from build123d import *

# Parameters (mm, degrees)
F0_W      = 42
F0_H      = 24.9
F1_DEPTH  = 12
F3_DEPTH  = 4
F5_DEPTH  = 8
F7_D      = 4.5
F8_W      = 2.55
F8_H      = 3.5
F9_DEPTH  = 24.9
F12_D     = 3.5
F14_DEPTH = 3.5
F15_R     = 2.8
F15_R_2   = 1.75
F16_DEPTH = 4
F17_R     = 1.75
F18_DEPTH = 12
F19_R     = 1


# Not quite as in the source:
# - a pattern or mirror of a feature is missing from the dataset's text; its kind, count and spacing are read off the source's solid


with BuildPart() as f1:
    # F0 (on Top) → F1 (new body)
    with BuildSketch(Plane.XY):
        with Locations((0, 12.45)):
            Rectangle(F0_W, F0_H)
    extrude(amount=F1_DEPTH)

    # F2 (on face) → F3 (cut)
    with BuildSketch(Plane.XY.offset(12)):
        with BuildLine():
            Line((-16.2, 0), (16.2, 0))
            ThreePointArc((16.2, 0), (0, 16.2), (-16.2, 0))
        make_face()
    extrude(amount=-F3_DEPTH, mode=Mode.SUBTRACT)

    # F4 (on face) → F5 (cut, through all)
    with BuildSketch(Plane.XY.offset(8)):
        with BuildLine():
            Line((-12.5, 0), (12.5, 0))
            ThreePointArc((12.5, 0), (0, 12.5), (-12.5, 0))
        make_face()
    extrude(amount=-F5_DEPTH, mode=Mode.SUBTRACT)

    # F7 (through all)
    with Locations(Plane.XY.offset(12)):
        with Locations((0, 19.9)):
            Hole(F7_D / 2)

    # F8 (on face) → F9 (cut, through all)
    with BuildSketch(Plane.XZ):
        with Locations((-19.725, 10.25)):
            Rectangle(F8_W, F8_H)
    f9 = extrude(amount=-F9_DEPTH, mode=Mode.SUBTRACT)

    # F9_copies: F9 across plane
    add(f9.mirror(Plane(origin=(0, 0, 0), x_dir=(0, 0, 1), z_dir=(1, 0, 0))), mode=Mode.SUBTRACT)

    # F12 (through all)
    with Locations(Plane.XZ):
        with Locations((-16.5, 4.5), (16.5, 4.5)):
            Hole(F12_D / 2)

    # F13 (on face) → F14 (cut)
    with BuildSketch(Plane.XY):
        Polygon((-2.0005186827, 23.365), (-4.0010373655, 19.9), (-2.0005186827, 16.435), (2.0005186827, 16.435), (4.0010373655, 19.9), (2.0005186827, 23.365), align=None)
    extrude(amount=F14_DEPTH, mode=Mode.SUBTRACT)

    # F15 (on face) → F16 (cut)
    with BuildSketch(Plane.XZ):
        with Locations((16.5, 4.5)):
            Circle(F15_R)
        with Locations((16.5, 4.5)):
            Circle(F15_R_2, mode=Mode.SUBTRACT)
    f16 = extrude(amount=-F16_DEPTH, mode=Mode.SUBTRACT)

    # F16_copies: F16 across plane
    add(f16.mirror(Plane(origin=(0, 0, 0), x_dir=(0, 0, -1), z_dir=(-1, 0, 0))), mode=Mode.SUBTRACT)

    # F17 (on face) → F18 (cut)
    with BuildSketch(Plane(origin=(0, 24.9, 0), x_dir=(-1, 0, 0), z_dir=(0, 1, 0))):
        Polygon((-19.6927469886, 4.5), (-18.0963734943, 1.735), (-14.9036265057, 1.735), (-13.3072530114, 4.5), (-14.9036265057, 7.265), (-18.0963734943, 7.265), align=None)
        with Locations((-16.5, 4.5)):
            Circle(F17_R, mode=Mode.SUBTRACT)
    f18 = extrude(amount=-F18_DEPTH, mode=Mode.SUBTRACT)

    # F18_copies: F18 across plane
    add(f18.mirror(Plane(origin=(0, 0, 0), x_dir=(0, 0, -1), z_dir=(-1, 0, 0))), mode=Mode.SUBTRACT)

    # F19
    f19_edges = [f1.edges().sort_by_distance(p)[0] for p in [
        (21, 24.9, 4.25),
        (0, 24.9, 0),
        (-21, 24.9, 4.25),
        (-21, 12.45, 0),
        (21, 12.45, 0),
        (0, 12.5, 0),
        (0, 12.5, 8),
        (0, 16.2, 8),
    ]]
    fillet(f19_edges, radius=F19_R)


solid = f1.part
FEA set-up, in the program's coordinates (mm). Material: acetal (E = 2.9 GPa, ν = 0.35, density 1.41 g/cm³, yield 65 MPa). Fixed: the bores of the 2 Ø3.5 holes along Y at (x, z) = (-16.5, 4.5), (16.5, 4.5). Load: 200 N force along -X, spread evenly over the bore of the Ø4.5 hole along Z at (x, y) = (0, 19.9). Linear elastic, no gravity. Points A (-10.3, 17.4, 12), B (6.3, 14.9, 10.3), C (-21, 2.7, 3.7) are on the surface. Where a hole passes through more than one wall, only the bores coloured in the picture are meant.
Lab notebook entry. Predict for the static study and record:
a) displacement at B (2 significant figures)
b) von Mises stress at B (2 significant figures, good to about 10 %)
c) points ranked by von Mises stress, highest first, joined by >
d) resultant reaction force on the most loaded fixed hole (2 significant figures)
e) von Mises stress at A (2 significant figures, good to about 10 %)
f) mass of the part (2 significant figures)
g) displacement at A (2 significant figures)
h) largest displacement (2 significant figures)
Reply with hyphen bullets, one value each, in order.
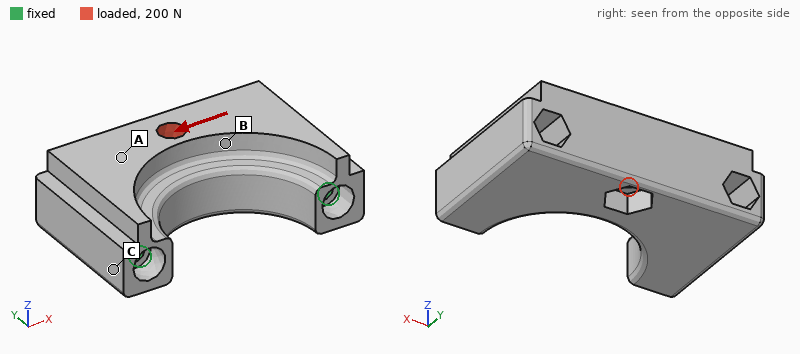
- 9.7 µm
- 2.0 MPa
- B > A > C
- 110 N
- 0.96 MPa
- 10 g
- 10 µm
- 16 µm
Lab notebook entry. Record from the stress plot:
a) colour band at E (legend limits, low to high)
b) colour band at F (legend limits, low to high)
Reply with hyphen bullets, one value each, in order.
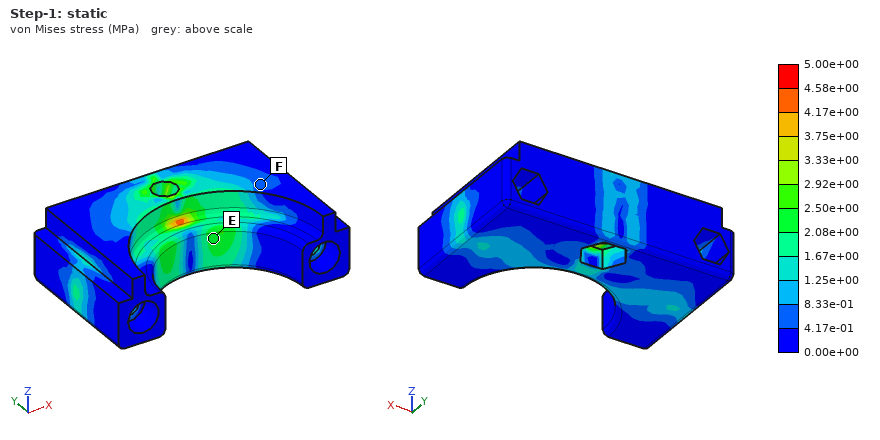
- 2.08e+00 to 2.50e+00 MPa
- 4.17e-01 to 8.33e-01 MPa
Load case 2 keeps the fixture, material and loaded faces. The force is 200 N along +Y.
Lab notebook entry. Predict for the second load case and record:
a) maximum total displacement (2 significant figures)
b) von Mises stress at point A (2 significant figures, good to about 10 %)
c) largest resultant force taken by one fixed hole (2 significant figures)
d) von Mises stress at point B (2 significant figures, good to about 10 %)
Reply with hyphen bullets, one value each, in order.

- 40 µm
- 1.7 MPa
- 130 N
- 2.0 MPa
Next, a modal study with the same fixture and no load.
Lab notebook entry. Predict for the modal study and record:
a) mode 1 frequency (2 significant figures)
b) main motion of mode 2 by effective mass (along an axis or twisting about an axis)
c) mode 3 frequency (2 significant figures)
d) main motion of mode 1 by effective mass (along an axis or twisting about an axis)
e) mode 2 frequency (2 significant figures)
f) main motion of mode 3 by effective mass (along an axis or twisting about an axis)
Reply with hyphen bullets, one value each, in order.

- 4000 Hz
- twisting about Y
- 8700 Hz
- along Z
- 7200 Hz
- along X
